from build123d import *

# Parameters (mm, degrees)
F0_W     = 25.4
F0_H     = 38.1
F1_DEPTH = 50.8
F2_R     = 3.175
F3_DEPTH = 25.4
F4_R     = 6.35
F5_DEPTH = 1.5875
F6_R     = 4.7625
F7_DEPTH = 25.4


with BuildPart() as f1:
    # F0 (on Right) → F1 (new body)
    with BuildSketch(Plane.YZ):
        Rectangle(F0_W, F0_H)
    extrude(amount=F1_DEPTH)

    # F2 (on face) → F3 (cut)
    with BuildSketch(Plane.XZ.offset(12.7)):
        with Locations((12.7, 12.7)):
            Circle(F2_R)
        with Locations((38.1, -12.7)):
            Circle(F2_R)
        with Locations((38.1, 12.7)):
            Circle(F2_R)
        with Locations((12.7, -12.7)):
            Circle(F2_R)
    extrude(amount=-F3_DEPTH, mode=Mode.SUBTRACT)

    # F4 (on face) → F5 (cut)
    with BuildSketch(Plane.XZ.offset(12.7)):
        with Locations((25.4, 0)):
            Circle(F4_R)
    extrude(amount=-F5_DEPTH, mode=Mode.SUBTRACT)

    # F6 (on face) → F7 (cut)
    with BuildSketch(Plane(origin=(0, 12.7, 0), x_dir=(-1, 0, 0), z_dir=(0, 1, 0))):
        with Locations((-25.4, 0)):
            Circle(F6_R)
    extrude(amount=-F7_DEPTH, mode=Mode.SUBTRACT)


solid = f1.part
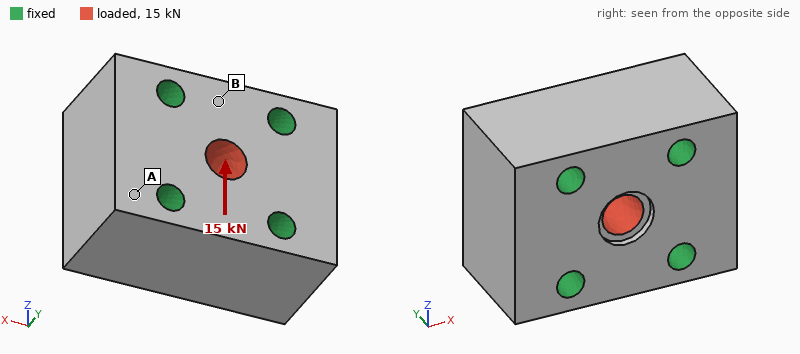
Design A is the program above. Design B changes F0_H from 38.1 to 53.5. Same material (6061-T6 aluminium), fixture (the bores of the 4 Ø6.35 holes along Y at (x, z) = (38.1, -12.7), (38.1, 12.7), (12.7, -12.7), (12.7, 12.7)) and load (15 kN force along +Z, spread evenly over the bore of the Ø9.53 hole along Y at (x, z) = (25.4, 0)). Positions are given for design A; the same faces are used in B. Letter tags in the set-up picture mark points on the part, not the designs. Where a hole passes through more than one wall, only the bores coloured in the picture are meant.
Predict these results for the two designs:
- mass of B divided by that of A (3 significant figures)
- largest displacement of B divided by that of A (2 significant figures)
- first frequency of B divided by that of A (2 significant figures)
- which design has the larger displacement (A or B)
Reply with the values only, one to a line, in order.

1.45
0.90
0.84
A
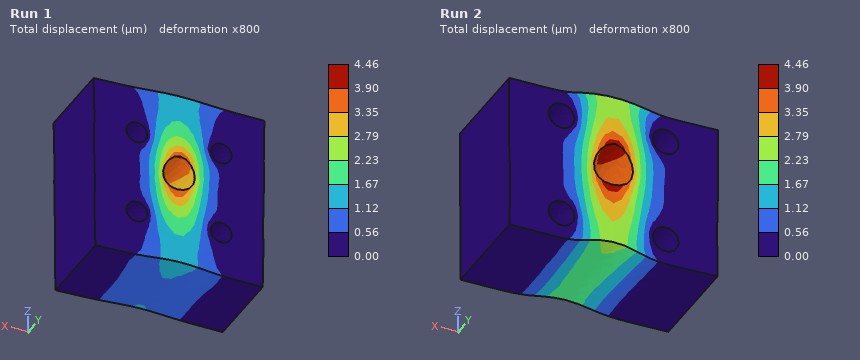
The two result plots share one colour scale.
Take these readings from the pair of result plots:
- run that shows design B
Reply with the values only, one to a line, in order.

Run 1
